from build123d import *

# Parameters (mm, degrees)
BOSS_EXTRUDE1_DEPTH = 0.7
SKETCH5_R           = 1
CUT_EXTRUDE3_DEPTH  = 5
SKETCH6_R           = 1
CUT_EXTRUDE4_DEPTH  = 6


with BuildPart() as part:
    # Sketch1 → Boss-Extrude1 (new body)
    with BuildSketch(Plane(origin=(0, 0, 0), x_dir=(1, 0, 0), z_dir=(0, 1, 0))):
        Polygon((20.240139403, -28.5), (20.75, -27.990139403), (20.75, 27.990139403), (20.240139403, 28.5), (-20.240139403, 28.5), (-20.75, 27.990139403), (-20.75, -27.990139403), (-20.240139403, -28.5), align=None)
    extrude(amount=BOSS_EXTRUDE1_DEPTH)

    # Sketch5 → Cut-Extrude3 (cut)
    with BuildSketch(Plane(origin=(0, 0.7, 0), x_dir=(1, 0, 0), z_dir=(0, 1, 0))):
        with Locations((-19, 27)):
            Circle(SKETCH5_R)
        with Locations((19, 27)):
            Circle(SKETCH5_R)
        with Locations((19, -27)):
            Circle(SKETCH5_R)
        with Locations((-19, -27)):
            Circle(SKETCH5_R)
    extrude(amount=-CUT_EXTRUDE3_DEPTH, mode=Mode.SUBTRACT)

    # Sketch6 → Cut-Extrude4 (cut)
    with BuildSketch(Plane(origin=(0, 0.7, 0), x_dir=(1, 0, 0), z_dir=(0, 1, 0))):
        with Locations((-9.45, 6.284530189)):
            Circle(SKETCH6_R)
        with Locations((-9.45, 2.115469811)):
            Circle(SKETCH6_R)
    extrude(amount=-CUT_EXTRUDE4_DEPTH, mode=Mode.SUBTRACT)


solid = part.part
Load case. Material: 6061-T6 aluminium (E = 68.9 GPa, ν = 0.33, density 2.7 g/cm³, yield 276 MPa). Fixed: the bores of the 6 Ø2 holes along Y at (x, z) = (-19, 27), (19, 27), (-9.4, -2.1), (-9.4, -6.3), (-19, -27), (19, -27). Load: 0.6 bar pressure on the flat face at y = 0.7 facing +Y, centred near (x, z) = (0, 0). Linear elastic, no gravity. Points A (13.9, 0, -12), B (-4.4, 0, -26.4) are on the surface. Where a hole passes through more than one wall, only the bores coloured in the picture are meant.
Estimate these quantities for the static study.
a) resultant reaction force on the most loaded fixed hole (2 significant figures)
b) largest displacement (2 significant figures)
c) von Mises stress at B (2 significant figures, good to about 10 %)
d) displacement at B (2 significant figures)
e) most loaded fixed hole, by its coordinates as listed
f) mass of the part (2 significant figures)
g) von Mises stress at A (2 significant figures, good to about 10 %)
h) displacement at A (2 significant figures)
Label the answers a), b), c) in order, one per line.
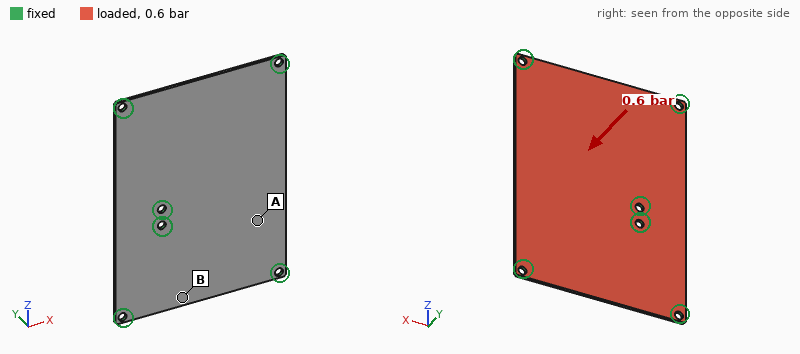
a) 40 N
b) 0.58 mm
c) 23 MPa
d) 0.10 mm
e) (-9.4, -2.1)
f) 4.4 g
g) 52 MPa
h) 0.32 mm
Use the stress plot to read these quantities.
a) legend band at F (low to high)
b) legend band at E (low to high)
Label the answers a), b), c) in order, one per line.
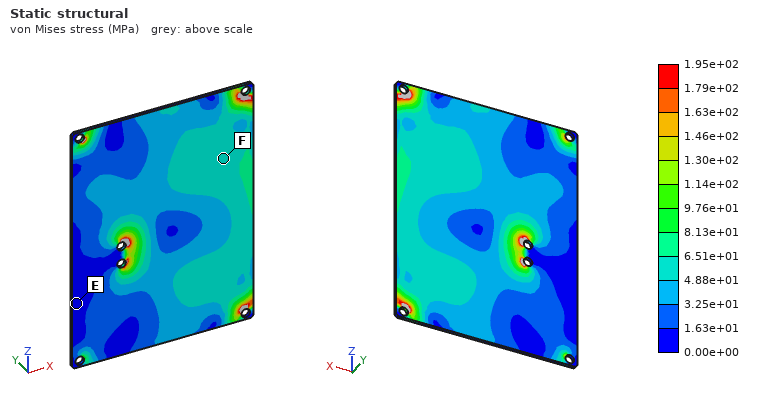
a) 4.88e+01 to 6.51e+01 MPa
b) 0.00e+00 to 1.63e+01 MPa
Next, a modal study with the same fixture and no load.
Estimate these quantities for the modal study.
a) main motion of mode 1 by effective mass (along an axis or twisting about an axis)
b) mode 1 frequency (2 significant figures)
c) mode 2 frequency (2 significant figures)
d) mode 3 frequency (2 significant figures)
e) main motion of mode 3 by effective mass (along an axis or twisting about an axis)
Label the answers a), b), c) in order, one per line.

a) along Y
b) 1600 Hz
c) 2500 Hz
d) 2900 Hz
e) along Y
